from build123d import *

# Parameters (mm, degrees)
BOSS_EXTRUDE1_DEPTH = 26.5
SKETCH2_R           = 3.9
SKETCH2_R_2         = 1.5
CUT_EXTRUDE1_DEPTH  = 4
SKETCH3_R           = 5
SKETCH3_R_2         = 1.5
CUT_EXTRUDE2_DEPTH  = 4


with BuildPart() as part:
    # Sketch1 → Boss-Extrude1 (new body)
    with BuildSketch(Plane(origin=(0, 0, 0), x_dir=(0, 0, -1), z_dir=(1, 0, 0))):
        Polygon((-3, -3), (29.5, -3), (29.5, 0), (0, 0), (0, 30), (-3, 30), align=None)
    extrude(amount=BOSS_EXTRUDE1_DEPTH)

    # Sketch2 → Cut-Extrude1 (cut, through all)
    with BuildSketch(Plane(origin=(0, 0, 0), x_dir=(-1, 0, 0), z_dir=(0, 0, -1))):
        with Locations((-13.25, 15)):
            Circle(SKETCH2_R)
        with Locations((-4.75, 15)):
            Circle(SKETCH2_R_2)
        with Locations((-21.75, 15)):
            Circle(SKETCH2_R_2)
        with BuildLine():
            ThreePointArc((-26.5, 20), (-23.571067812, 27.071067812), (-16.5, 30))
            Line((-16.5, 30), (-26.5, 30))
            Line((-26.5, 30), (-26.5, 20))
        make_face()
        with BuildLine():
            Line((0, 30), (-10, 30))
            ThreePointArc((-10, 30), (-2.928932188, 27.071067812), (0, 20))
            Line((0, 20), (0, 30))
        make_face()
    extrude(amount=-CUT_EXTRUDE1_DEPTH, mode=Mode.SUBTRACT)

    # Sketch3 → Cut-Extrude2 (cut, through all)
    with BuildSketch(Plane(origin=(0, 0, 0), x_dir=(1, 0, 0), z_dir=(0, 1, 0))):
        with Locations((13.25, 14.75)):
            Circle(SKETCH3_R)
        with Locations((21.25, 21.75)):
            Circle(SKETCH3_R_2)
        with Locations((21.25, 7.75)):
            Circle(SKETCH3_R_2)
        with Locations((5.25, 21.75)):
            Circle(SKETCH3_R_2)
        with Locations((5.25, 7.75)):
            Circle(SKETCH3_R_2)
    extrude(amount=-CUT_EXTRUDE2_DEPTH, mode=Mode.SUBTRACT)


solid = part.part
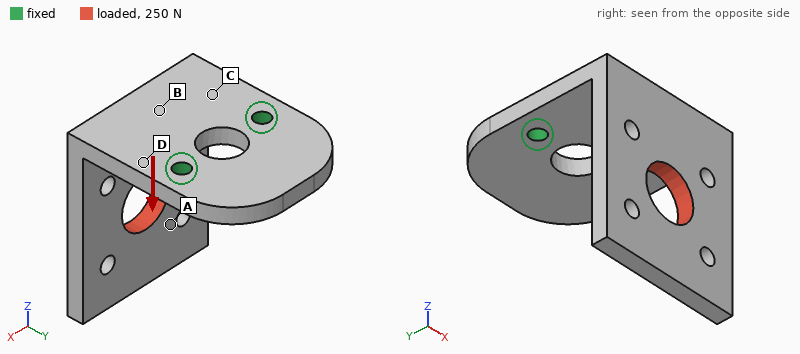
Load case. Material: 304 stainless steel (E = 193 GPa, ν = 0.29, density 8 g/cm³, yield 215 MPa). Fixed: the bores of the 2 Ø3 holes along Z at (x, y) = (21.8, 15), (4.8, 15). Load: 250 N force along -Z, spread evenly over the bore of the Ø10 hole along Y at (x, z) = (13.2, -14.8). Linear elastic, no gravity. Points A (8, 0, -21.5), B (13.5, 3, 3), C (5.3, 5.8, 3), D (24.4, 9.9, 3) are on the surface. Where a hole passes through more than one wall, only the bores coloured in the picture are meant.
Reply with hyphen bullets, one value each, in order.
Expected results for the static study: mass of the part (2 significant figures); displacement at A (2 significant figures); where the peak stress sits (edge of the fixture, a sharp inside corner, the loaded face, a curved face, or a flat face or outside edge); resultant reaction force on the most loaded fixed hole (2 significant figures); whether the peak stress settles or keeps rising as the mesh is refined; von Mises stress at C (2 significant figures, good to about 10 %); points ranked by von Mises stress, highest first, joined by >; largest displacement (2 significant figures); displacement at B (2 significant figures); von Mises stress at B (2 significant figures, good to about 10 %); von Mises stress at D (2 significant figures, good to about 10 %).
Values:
- 35 g
- 0.080 mm
- edge of the fixture
- 130 N
- keeps rising
- 45 MPa
- D > C > B > A
- 0.11 mm
- 0.023 mm
- 25 MPa
- 84 MPa
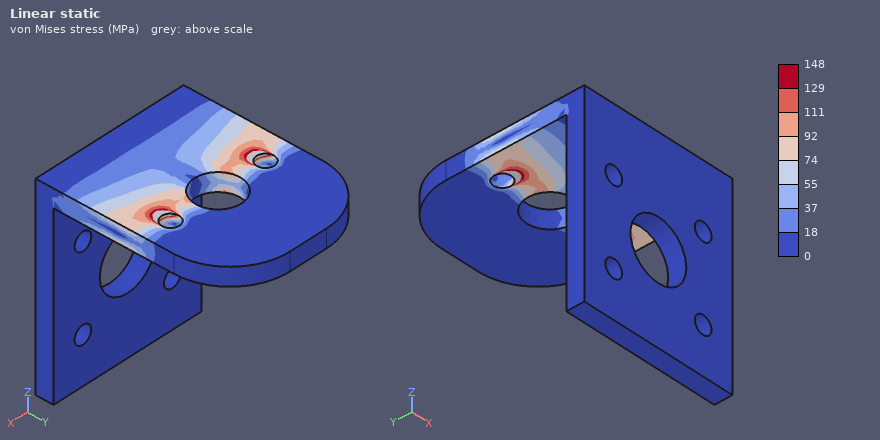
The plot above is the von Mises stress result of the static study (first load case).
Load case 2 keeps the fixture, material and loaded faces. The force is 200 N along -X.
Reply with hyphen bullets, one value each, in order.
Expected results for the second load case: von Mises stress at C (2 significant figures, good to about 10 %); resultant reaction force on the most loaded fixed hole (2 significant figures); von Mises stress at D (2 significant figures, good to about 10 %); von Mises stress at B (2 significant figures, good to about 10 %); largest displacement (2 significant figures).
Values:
- 40 MPa
- 250 N
- 47 MPa
- 37 MPa
- 55 µm
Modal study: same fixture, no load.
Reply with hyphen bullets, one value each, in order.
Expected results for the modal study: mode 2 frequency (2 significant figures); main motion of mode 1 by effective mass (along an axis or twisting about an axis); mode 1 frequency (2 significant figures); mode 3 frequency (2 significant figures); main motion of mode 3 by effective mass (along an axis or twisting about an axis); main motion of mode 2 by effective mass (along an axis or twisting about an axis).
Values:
- 2700 Hz
- along Y
- 1400 Hz
- 4300 Hz
- along Z
- along X
